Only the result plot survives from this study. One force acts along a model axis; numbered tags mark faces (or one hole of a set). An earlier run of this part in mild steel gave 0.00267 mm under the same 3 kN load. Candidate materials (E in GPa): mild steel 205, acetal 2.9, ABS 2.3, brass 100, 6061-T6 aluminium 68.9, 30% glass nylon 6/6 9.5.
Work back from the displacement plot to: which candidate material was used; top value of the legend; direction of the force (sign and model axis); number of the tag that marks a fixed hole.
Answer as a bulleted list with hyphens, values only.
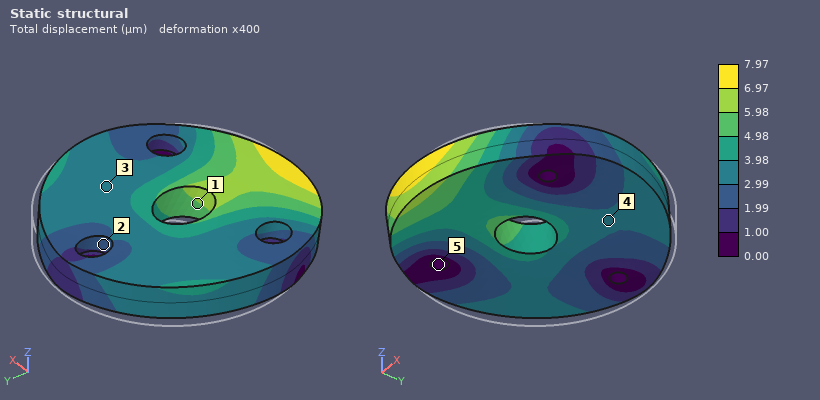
- 6061-T6 aluminium
- 7.97 µm
- -Y
- 5
